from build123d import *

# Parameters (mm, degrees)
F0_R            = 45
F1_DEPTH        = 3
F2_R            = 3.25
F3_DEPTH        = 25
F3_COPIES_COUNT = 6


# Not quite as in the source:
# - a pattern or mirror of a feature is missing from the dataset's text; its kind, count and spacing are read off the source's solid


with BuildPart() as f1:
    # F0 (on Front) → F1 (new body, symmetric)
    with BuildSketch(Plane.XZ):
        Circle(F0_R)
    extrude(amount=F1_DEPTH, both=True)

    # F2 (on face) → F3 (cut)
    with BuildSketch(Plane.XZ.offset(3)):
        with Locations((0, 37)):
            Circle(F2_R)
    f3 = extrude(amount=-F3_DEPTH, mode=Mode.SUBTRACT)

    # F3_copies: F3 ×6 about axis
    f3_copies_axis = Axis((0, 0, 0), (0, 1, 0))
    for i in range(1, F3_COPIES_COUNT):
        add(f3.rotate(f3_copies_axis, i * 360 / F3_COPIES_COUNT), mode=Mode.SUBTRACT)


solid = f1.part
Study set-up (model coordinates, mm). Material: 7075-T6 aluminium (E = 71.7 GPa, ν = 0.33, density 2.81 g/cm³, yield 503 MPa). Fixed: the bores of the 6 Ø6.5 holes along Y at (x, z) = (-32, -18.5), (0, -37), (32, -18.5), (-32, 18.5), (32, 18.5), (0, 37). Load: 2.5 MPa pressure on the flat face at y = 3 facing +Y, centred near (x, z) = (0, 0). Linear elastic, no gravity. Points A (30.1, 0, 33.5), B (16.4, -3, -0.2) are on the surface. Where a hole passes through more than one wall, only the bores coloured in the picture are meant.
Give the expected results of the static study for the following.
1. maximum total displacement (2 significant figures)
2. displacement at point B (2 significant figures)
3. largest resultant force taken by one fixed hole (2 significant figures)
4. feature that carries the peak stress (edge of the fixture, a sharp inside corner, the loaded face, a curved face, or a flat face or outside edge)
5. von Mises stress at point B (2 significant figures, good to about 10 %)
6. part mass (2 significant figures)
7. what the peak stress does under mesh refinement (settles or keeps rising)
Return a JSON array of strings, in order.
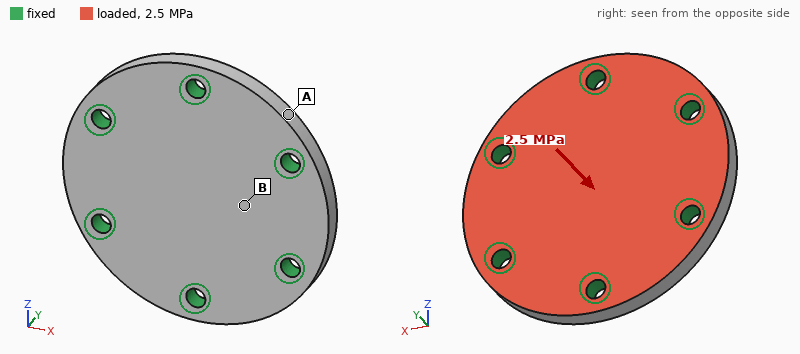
["61 µm", "43 µm", "2.6 kN", "edge of the fixture", "32 MPa", "100 g", "keeps rising"]
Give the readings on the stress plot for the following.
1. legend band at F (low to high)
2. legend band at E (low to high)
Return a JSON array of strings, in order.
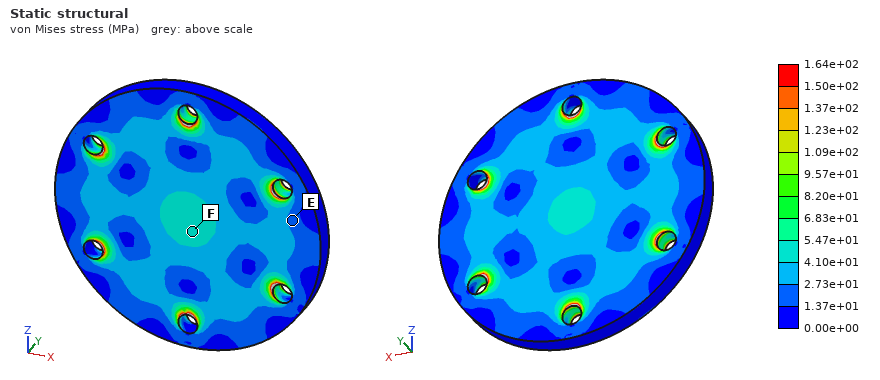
["4.10e+01 to 5.47e+01 MPa", "1.37e+01 to 2.73e+01 MPa"]
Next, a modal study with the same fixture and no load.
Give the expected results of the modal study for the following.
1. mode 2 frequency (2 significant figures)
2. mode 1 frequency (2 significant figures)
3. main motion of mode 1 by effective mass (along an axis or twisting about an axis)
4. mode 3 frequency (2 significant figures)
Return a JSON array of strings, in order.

["18 kHz", "9500 Hz", "along Y", "18 kHz"]
